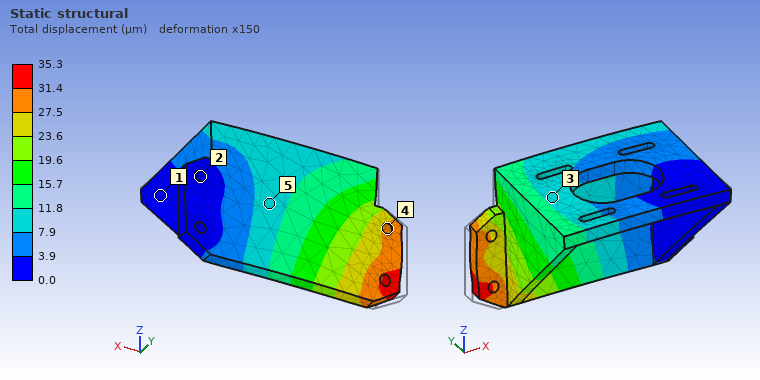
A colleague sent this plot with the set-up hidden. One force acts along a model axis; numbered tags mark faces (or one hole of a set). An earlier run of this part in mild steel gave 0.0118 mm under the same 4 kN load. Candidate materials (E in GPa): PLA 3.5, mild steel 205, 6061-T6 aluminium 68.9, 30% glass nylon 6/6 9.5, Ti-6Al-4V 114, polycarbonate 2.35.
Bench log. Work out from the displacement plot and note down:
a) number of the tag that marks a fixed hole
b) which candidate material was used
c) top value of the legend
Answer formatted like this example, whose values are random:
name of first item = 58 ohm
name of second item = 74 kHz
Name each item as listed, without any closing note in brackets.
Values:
number of the tag that marks a fixed hole = 2
which candidate material was used = 6061-T6 aluminium
top value of the legend = 35.3 µm
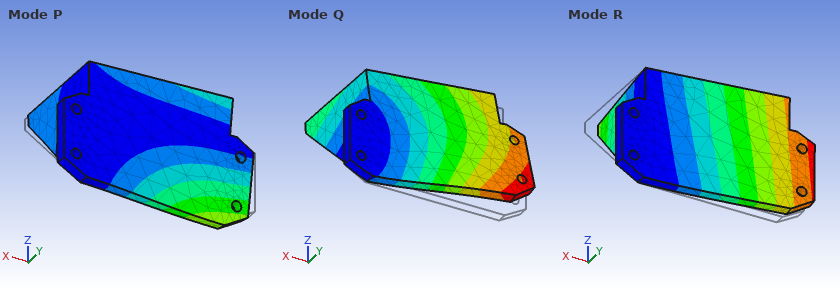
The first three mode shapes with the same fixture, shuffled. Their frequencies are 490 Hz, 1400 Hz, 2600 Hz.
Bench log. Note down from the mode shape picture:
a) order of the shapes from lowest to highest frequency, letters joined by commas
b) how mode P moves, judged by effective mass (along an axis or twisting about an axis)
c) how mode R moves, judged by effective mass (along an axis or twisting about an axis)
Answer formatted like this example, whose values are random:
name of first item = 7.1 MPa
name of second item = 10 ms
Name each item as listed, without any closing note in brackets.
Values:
order of the shapes from lowest to highest frequency, letters joined by commas = R, P, Q
how mode P moves, judged by effective mass = along Z
how mode R moves, judged by effective mass = along Y
